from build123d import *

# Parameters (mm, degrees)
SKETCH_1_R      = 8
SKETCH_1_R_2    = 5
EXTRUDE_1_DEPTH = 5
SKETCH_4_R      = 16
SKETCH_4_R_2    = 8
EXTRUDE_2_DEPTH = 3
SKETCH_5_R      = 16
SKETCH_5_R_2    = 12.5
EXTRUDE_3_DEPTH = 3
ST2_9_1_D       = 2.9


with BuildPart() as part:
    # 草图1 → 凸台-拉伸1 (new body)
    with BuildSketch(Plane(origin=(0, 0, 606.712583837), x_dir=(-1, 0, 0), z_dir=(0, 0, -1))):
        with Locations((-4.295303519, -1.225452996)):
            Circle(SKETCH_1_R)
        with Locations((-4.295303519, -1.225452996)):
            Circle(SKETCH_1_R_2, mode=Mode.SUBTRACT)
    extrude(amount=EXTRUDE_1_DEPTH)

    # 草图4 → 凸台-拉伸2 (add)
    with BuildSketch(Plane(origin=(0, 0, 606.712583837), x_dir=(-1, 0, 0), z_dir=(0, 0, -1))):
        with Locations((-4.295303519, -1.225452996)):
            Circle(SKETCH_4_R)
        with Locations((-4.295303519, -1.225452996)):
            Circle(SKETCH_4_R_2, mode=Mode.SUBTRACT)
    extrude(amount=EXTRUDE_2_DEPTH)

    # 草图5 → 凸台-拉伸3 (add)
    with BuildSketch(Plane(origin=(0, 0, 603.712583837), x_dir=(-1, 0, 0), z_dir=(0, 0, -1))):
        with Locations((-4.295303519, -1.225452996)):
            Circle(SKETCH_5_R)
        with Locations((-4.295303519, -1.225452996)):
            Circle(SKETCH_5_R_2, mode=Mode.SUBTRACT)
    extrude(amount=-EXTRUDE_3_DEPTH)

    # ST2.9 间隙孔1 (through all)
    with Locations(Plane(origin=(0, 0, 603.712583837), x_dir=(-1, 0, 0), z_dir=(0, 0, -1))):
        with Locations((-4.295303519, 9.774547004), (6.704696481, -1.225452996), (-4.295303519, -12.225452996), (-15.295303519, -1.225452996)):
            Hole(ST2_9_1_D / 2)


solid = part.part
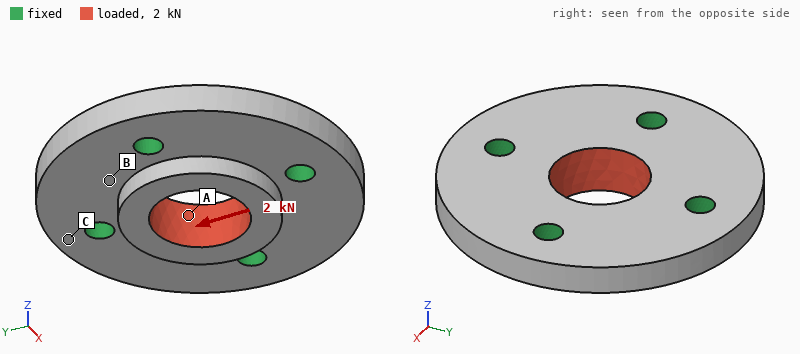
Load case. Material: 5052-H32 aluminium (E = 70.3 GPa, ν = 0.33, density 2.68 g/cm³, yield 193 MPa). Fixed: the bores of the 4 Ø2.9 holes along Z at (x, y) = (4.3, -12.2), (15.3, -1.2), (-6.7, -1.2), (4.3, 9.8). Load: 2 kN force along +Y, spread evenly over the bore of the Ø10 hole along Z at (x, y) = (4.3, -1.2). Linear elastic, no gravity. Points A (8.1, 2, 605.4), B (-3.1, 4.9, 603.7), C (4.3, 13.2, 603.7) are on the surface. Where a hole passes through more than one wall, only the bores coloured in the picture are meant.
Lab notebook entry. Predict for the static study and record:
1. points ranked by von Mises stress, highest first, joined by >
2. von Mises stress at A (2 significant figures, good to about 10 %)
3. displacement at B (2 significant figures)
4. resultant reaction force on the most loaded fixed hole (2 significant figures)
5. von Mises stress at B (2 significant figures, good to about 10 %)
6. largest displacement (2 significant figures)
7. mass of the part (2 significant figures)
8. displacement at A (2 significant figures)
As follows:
A > B > C
22 MPa
1.6 µm
600 N
10 MPa
3.5 µm
6.3 g
2.4 µm
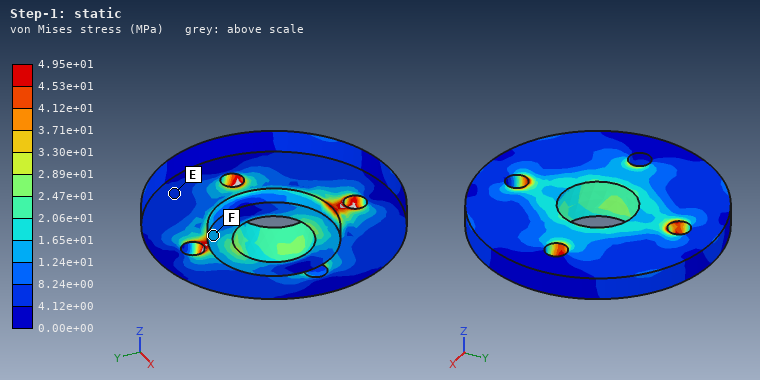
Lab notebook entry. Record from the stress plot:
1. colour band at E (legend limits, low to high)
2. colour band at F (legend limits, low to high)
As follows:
4.12e+00 to 8.24e+00 MPa
1.24e+01 to 1.65e+01 MPa
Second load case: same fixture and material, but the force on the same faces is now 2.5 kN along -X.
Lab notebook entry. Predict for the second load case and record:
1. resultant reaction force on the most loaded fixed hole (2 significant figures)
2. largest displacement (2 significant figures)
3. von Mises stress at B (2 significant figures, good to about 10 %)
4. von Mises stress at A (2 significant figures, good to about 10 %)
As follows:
750 N
4.4 µm
14 MPa
26 MPa
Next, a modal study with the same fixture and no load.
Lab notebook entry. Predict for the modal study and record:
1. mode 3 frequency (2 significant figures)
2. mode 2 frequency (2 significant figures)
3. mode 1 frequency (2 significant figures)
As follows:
37 kHz
37 kHz
35 kHz
